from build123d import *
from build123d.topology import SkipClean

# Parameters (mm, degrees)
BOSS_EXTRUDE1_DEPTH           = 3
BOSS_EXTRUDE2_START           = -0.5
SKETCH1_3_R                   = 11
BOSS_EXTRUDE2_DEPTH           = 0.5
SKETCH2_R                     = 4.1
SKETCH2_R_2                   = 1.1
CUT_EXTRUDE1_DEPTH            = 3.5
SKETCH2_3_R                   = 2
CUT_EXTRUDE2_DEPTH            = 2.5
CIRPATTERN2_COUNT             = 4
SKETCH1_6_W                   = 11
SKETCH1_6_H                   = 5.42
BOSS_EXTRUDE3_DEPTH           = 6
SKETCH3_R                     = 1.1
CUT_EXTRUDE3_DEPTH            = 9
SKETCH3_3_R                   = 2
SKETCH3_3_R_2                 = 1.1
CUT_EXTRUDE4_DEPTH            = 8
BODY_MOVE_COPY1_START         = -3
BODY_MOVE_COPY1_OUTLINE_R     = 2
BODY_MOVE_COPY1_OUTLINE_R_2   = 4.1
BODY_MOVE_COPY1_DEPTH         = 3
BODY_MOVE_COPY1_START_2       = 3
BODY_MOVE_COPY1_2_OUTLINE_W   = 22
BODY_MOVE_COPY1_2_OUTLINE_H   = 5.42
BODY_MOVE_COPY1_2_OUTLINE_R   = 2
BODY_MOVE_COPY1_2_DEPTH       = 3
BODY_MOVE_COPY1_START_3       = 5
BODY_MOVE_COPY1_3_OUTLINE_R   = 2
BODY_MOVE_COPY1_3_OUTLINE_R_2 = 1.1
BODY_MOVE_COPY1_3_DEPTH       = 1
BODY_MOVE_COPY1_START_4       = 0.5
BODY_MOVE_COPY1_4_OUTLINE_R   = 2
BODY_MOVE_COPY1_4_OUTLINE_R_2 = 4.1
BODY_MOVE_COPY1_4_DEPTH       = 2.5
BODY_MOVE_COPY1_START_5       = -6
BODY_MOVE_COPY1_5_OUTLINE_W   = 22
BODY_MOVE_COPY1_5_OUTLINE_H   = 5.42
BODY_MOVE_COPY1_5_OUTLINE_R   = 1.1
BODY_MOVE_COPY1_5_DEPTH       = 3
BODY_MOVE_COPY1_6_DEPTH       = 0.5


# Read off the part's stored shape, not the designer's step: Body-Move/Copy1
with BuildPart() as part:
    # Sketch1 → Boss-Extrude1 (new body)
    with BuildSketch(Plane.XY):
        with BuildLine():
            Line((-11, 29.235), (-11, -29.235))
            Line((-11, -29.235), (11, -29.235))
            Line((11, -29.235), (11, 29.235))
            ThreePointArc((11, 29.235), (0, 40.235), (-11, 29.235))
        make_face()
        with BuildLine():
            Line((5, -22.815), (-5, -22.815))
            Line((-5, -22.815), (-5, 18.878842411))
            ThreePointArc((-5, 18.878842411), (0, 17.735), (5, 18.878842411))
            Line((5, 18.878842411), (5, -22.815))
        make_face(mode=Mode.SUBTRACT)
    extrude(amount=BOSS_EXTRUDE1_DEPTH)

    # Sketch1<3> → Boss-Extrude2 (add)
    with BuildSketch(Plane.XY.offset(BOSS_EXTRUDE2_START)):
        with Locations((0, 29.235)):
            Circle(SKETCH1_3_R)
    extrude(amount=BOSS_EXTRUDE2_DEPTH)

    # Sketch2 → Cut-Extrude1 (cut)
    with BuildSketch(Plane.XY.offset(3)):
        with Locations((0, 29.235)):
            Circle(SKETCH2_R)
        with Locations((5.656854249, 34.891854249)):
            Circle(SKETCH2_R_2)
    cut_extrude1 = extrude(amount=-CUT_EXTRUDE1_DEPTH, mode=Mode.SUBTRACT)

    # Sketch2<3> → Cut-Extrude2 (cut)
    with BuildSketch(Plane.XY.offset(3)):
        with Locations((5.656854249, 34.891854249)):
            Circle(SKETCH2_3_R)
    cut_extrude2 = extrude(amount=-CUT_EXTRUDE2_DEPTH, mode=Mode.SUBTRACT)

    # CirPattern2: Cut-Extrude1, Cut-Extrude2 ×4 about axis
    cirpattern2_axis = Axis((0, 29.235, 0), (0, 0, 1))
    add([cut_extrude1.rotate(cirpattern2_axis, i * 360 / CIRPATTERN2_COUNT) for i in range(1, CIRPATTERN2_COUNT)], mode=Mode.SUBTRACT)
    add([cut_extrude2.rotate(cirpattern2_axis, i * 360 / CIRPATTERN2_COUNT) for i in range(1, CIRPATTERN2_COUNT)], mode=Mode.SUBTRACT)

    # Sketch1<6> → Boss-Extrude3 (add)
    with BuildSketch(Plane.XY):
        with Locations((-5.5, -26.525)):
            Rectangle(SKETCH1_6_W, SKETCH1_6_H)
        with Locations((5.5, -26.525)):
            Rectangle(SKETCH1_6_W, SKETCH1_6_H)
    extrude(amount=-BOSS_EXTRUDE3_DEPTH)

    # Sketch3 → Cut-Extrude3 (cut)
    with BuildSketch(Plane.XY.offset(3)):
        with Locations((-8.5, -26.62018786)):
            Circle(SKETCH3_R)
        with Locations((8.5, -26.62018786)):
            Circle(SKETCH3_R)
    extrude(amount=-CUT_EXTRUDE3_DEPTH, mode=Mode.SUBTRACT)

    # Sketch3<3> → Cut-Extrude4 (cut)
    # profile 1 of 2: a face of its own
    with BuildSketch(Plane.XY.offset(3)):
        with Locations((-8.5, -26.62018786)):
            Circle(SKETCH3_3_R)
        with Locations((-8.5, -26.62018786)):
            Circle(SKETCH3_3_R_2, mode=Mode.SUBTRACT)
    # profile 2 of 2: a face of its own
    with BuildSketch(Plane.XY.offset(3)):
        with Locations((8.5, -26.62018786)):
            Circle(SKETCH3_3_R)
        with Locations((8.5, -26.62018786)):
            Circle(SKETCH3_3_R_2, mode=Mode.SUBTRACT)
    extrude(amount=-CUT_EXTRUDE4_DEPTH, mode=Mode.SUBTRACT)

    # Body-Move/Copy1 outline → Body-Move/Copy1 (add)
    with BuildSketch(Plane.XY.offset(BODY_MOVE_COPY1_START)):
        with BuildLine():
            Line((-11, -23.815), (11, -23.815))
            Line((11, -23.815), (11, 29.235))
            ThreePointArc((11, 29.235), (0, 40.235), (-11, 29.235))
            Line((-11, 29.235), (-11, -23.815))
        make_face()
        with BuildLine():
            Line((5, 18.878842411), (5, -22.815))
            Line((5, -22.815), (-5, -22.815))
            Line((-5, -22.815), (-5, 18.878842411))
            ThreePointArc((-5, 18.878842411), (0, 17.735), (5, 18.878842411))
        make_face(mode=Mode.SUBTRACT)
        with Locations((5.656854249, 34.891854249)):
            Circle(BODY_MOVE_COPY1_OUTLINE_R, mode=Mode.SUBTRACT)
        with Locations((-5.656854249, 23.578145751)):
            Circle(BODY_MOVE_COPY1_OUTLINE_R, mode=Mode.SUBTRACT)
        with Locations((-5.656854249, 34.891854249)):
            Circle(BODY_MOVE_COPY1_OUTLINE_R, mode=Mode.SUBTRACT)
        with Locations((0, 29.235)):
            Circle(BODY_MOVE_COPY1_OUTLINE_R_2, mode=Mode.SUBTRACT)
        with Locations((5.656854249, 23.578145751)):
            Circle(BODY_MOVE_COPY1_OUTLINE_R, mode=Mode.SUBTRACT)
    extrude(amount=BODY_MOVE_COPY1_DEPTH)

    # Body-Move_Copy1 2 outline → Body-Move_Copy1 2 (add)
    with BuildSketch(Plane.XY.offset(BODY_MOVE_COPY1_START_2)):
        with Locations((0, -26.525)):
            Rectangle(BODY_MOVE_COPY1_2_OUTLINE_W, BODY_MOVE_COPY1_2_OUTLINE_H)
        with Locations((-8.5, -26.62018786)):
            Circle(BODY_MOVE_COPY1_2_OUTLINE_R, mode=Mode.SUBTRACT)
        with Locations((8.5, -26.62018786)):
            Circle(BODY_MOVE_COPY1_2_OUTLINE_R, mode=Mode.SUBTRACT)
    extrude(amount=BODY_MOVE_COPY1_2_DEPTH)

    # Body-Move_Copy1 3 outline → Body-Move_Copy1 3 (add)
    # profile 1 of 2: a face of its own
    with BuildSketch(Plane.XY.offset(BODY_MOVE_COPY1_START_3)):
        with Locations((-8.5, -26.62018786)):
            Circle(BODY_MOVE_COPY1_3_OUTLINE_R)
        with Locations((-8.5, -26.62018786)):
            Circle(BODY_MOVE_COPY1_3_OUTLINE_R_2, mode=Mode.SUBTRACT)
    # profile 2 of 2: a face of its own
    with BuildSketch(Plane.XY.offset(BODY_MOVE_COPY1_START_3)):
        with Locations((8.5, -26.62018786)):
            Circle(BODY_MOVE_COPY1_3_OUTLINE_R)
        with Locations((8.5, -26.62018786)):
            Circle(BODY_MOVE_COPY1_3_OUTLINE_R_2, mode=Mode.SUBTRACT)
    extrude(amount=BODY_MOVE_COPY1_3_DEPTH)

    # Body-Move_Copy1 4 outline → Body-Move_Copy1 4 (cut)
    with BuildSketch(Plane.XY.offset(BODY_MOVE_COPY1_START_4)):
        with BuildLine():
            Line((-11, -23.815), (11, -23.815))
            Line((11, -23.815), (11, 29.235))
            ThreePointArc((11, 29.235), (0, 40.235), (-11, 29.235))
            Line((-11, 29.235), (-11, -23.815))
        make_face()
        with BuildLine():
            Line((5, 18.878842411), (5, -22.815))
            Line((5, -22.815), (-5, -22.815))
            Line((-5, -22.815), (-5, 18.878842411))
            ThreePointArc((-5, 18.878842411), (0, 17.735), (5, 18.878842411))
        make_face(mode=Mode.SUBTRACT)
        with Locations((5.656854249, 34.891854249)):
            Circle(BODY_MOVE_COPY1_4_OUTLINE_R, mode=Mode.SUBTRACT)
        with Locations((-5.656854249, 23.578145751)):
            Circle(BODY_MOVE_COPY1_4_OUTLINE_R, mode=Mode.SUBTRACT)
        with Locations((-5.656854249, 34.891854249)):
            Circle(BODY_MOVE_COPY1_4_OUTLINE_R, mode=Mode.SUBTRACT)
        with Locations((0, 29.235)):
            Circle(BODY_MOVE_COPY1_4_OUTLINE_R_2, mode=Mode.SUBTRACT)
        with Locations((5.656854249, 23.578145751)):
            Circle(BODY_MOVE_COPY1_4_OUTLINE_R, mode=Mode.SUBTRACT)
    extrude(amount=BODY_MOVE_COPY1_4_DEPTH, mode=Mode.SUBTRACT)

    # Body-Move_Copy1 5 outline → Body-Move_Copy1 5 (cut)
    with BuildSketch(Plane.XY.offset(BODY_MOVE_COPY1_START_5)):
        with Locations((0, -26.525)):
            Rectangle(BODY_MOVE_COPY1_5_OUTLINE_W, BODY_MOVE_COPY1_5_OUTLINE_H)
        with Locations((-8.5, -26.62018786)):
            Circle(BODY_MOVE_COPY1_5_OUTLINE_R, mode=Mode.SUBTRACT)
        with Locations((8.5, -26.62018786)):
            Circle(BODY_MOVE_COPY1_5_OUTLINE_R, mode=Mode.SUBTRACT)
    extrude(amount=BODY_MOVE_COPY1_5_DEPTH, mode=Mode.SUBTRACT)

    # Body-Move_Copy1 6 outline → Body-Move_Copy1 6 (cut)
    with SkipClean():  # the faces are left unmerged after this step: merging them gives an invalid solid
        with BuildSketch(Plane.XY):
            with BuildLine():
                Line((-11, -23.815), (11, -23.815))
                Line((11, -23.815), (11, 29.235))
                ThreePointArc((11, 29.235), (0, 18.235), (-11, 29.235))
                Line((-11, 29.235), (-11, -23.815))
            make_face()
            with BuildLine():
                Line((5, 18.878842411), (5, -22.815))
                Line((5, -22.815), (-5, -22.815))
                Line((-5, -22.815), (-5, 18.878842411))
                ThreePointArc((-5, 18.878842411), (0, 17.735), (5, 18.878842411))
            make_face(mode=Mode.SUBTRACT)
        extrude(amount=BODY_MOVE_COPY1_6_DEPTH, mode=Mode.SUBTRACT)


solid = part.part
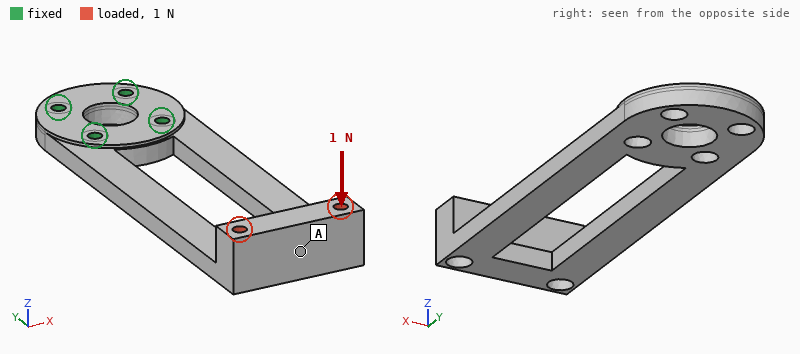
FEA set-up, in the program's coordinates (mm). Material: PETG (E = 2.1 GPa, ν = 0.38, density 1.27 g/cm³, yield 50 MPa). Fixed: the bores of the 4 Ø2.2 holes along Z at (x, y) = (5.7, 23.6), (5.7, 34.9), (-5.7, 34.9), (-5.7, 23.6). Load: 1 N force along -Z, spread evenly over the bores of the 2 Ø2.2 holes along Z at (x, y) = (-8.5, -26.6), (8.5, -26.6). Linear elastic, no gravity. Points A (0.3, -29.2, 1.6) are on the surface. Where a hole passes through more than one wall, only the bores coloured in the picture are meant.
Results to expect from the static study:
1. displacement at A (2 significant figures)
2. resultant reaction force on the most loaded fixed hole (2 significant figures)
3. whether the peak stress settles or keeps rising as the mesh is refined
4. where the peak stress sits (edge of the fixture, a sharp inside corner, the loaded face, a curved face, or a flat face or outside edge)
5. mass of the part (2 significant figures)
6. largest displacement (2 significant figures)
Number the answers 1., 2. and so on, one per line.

1. 0.81 mm
2. 4.0 N
3. keeps rising
4. edge of the fixture
5. 4.5 g
6. 0.82 mm
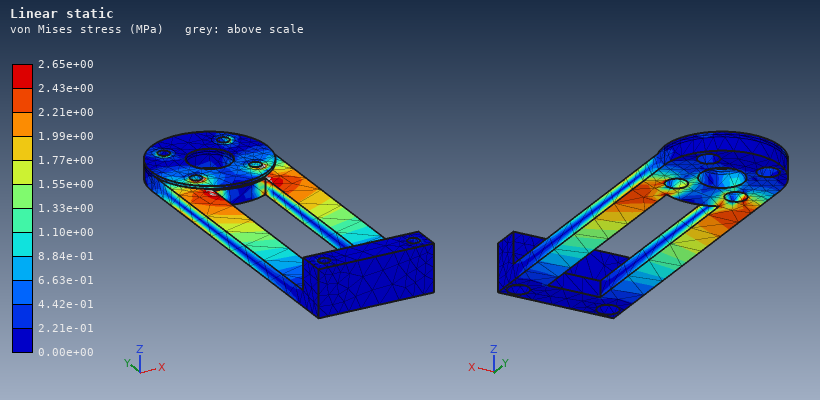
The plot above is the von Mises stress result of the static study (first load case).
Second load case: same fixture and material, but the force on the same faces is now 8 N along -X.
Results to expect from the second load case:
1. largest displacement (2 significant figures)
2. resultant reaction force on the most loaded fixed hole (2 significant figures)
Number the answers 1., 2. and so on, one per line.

1. 0.86 mm
2. 14 N
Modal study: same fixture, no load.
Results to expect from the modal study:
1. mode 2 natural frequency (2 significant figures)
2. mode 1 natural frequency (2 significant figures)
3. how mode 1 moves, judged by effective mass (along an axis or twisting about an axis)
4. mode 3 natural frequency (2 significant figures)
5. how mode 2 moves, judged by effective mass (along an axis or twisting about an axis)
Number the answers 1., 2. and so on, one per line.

1. 470 Hz
2. 150 Hz
3. along Z
4. 650 Hz
5. along X
